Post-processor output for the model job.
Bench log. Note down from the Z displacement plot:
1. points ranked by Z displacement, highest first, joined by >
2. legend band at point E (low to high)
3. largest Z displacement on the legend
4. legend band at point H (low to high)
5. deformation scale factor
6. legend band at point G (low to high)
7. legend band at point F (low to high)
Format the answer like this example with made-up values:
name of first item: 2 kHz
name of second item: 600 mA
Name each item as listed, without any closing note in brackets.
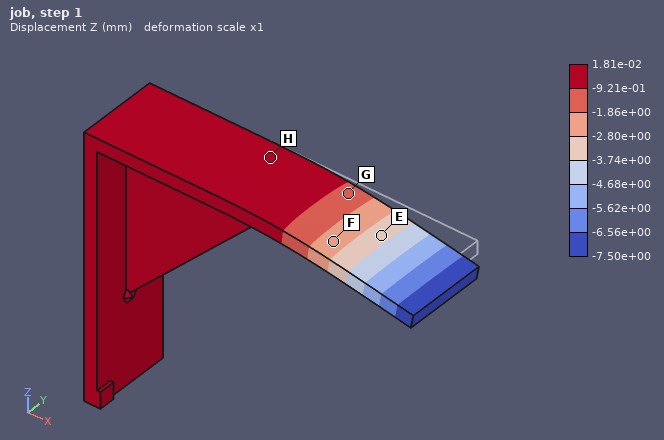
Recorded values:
points ranked by Z displacement, highest first, joined by >: H > G > F > E
legend band at point E: -3.74e+00 to -2.80e+00 mm
largest Z displacement on the legend: 1.81e-02 mm
legend band at point H: -9.21e-01 to 1.81e-02 mm
deformation scale factor: 1
legend band at point G: -1.86e+00 to -9.21e-01 mm
legend band at point F: -2.80e+00 to -1.86e+00 mm
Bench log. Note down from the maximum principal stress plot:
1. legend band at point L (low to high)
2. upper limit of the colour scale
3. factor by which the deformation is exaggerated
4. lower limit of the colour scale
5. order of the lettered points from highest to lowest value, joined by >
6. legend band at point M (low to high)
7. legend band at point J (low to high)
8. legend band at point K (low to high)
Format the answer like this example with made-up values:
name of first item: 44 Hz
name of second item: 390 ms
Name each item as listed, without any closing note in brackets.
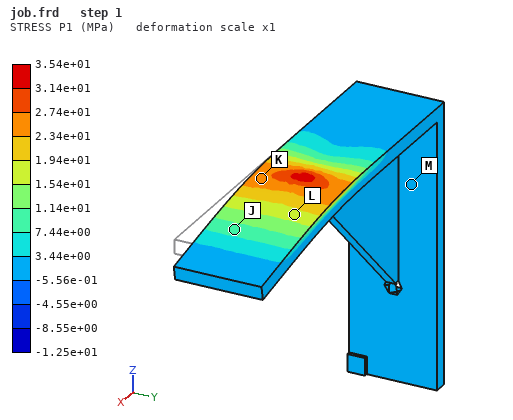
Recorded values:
legend band at point L: 1.54e+01 to 1.94e+01 MPa
upper limit of the colour scale: 3.54e+01 MPa
factor by which the deformation is exaggerated: 1
lower limit of the colour scale: -1.25e+01 MPa
order of the lettered points from highest to lowest value, joined by >: K > L > J > M
legend band at point M: -5.56e-01 to 3.44e+00 MPa
legend band at point J: 7.44e+00 to 1.14e+01 MPa
legend band at point K: 2.34e+01 to 2.74e+01 MPa
